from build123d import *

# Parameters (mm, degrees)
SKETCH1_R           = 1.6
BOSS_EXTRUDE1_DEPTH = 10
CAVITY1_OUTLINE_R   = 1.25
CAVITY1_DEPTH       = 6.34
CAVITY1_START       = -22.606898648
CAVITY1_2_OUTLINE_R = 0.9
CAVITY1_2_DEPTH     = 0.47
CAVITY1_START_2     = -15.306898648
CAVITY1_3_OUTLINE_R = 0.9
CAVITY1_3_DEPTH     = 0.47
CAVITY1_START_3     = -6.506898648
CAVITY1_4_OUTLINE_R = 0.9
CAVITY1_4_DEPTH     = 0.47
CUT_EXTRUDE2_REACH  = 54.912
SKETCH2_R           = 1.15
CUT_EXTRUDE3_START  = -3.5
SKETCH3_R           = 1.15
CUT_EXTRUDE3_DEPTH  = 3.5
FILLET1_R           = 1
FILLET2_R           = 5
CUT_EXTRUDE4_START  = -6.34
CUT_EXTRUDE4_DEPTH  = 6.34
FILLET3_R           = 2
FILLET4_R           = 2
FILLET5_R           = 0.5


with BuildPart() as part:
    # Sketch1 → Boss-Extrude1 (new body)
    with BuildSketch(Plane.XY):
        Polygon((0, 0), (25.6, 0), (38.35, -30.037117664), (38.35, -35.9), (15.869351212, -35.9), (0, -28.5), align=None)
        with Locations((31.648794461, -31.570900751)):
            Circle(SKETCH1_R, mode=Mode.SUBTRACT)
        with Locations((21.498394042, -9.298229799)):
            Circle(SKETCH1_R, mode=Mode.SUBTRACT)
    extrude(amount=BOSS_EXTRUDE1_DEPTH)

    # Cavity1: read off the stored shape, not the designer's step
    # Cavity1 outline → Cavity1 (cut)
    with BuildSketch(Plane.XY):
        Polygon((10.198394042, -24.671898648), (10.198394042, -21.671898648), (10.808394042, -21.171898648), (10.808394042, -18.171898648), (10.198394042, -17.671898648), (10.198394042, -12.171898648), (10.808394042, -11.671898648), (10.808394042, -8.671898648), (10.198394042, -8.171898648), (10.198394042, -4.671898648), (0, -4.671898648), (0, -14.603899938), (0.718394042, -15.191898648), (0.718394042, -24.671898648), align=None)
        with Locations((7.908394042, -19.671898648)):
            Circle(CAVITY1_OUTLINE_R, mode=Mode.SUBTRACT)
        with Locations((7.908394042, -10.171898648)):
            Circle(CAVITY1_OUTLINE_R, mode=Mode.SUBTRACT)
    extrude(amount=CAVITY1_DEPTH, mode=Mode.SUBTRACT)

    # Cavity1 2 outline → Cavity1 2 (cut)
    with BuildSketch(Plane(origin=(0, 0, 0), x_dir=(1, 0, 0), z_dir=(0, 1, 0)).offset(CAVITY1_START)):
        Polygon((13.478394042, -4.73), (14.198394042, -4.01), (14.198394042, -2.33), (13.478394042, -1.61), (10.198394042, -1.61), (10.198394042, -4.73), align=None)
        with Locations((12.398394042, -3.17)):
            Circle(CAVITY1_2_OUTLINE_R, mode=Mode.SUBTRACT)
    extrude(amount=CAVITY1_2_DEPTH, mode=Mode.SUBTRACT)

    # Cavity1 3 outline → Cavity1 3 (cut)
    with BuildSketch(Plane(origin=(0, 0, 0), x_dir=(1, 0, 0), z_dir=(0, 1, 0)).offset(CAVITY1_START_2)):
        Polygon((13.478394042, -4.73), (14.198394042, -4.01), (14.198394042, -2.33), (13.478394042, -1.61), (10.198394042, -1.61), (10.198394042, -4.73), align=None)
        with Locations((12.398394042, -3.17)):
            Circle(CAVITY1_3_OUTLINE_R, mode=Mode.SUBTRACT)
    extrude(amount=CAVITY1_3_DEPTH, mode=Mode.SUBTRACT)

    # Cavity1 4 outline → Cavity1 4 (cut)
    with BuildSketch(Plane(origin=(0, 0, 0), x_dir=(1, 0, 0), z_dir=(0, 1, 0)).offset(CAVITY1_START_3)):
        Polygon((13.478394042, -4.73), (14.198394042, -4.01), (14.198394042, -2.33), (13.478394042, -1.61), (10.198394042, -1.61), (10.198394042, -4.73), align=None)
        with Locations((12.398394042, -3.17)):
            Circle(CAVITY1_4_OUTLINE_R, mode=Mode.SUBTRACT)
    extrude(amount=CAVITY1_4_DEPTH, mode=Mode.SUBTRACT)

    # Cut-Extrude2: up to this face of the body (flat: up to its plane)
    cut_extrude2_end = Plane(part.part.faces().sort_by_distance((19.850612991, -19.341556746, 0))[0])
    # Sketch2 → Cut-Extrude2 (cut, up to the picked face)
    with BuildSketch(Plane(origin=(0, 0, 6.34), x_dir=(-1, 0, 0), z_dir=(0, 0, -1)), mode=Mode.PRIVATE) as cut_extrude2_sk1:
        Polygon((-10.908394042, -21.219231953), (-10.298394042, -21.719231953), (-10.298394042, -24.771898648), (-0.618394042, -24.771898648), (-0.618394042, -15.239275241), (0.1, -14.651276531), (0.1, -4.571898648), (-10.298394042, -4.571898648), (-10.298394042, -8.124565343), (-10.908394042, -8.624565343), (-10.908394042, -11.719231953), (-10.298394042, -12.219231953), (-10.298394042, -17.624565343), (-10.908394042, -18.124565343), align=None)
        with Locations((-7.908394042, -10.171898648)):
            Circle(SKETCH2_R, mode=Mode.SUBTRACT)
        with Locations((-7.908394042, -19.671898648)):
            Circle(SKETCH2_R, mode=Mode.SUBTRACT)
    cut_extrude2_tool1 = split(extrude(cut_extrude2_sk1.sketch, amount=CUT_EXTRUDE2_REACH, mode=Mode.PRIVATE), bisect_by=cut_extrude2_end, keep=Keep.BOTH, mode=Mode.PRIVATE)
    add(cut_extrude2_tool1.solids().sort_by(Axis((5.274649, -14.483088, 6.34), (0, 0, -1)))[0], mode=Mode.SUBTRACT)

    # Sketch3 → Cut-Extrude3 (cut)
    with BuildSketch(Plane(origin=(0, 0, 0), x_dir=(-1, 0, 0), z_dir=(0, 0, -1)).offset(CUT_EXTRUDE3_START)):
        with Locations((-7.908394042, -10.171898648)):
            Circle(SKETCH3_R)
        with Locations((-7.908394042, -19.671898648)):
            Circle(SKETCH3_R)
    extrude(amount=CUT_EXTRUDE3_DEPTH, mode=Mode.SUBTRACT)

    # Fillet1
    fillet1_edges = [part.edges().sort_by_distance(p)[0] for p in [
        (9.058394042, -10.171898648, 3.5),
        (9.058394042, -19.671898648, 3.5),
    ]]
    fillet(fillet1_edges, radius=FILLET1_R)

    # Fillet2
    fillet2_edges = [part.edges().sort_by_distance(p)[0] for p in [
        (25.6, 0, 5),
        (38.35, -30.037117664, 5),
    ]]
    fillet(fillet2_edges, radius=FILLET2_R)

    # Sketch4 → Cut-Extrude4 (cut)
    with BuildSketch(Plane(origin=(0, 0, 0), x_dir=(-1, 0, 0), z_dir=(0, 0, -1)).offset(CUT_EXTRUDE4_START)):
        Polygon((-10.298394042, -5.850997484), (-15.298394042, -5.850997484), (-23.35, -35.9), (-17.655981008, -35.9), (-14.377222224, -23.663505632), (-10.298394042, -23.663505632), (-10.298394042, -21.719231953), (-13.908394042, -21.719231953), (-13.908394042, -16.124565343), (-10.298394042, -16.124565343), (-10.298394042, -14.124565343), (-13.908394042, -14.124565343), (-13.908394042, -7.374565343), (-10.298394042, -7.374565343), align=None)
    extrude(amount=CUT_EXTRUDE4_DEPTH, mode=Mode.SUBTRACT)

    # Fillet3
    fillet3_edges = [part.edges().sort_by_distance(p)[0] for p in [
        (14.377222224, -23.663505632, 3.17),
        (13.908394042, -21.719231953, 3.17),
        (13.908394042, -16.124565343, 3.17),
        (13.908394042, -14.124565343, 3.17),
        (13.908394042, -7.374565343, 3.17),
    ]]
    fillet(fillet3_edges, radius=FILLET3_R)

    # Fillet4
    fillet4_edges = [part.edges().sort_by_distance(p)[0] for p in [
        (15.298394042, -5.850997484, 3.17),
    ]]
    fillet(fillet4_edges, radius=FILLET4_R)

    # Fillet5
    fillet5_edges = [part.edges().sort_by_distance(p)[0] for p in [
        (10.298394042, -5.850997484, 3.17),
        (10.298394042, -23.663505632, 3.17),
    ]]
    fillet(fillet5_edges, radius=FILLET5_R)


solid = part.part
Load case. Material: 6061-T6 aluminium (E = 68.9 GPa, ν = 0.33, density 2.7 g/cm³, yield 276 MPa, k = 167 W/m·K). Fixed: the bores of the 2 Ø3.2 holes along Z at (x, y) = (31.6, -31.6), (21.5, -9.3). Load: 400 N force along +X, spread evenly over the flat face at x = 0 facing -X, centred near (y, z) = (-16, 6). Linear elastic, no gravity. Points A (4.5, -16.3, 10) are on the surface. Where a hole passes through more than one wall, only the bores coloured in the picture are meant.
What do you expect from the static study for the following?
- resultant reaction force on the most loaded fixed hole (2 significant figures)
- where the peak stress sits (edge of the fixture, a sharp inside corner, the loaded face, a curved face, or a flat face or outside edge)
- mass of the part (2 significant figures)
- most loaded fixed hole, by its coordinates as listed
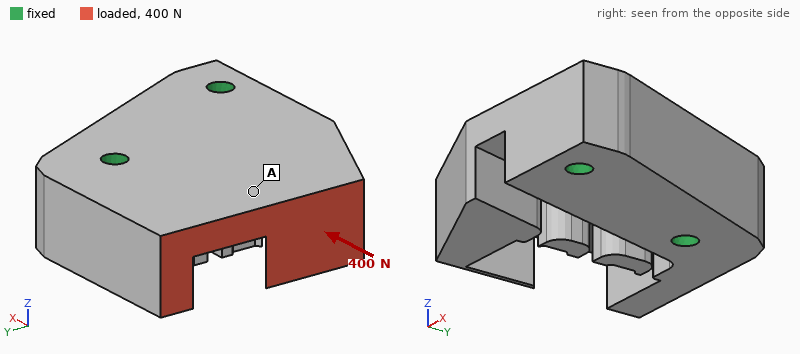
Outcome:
270 N
the loaded face
24 g
(21.5, -9.3)
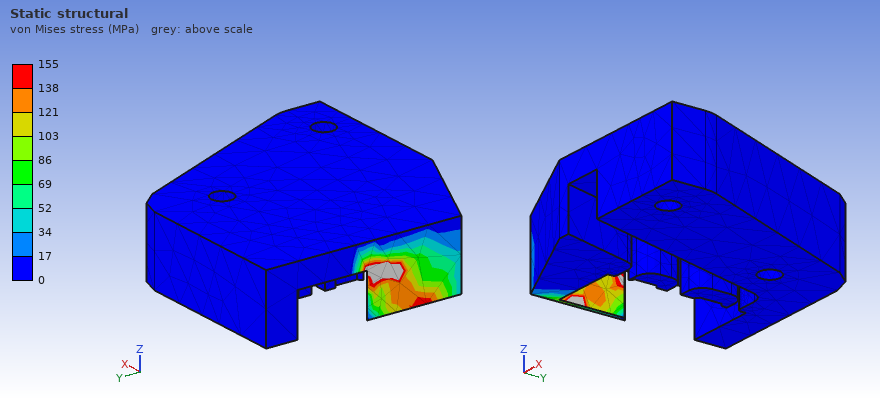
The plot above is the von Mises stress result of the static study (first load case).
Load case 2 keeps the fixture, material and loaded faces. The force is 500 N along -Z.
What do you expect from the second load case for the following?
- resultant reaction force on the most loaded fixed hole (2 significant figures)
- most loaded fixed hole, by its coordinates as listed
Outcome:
470 N
(21.5, -9.3)
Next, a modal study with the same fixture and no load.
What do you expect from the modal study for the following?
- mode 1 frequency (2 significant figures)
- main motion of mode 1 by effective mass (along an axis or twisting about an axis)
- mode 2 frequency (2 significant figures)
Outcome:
6600 Hz
along Z
14 kHz
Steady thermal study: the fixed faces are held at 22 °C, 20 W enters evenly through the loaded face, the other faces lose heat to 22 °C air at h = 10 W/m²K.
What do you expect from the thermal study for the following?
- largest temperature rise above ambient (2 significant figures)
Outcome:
36 K
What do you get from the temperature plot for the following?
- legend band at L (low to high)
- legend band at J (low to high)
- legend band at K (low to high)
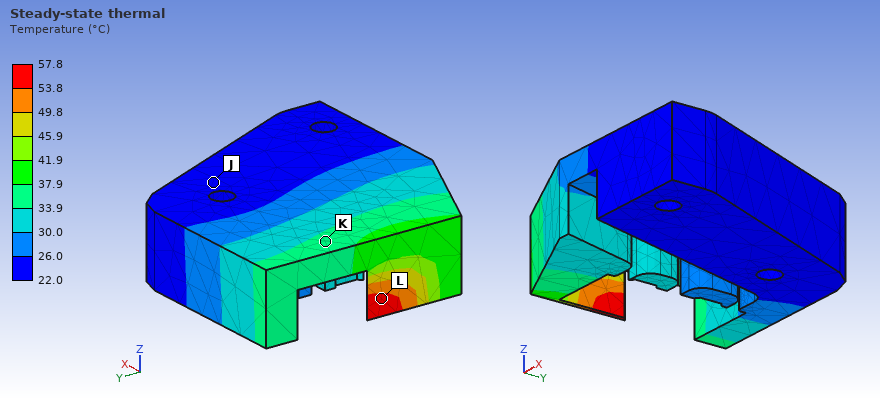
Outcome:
53.8 to 57.8 °C
22.0 to 26.0 °C
33.9 to 37.9 °C
